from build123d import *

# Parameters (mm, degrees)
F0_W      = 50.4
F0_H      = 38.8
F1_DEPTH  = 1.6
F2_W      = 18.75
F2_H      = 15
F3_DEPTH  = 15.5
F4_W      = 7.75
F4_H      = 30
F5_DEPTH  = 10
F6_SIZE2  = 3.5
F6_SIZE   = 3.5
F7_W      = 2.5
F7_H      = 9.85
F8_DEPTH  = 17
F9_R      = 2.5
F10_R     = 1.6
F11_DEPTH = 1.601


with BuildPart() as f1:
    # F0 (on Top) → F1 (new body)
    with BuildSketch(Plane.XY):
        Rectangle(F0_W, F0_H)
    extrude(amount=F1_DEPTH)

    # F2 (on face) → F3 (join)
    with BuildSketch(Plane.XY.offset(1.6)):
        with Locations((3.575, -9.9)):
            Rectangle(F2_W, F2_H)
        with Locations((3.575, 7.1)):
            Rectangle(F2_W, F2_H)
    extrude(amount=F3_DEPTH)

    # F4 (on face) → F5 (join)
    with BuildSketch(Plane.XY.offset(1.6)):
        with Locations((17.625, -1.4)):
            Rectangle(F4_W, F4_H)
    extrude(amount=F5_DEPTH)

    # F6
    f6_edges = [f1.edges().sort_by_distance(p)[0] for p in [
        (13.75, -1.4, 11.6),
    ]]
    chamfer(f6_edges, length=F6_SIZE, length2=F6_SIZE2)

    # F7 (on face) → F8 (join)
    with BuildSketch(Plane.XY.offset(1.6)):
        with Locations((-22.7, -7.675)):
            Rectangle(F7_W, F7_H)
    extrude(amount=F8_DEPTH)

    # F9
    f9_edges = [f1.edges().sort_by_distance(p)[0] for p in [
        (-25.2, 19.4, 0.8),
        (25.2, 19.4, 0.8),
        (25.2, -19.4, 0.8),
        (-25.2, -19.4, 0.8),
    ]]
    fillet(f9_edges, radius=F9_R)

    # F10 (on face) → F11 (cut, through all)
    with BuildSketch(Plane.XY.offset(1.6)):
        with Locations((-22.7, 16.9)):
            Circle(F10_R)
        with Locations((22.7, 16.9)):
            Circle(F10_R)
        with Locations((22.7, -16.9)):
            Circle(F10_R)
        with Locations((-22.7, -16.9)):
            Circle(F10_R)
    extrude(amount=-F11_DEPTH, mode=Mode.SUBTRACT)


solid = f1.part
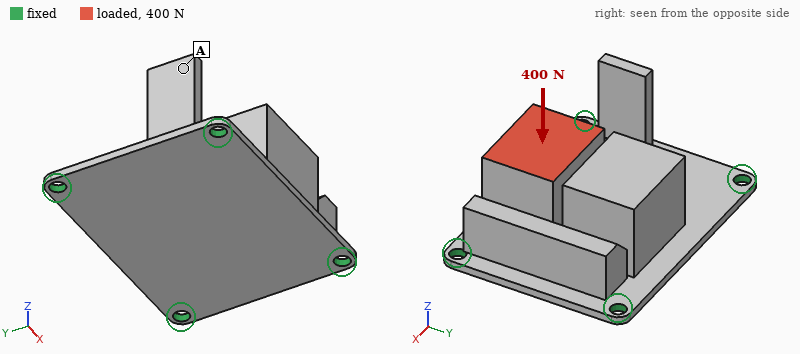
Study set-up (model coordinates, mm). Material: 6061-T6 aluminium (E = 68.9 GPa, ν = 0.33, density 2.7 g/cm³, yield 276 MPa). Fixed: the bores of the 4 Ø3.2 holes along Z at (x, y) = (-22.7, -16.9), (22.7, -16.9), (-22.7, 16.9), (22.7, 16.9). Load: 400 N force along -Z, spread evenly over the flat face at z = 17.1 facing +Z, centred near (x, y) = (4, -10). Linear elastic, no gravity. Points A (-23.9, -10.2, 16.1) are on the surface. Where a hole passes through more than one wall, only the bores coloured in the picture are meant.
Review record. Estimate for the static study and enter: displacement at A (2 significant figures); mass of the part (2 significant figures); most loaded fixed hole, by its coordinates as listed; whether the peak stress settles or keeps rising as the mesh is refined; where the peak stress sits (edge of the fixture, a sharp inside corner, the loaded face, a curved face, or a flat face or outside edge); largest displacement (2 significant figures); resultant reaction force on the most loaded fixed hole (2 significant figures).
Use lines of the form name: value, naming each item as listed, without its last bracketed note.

displacement at A: 0.075 mm
mass of the part: 39 g
most loaded fixed hole, by its coordinates as listed: (22.7, -16.9)
whether the peak stress settles or keeps rising as the mesh is refined: keeps rising
where the peak stress sits: edge of the fixture
largest displacement: 0.11 mm
resultant reaction force on the most loaded fixed hole: 250 N
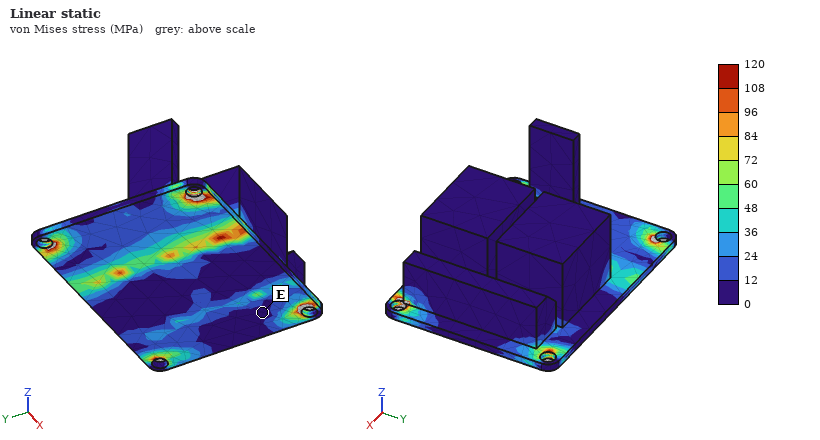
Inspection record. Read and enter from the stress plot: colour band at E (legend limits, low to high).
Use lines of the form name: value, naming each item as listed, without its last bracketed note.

colour band at E: 0 to 12 MPa
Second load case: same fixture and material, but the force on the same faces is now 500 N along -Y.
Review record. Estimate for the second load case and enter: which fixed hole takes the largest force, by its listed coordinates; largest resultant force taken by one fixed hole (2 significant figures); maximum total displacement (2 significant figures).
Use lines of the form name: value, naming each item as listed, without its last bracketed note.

which fixed hole takes the largest force, by its listed coordinates: (22.7, 16.9)
largest resultant force taken by one fixed hole: 410 N
maximum total displacement: 79 µm
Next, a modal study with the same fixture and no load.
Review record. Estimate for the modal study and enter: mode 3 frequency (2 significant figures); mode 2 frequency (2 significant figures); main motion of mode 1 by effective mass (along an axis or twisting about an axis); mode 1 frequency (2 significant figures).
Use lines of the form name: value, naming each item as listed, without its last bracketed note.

mode 3 frequency: 4500 Hz
mode 2 frequency: 4000 Hz
main motion of mode 1 by effective mass: along Z
mode 1 frequency: 2000 Hz
